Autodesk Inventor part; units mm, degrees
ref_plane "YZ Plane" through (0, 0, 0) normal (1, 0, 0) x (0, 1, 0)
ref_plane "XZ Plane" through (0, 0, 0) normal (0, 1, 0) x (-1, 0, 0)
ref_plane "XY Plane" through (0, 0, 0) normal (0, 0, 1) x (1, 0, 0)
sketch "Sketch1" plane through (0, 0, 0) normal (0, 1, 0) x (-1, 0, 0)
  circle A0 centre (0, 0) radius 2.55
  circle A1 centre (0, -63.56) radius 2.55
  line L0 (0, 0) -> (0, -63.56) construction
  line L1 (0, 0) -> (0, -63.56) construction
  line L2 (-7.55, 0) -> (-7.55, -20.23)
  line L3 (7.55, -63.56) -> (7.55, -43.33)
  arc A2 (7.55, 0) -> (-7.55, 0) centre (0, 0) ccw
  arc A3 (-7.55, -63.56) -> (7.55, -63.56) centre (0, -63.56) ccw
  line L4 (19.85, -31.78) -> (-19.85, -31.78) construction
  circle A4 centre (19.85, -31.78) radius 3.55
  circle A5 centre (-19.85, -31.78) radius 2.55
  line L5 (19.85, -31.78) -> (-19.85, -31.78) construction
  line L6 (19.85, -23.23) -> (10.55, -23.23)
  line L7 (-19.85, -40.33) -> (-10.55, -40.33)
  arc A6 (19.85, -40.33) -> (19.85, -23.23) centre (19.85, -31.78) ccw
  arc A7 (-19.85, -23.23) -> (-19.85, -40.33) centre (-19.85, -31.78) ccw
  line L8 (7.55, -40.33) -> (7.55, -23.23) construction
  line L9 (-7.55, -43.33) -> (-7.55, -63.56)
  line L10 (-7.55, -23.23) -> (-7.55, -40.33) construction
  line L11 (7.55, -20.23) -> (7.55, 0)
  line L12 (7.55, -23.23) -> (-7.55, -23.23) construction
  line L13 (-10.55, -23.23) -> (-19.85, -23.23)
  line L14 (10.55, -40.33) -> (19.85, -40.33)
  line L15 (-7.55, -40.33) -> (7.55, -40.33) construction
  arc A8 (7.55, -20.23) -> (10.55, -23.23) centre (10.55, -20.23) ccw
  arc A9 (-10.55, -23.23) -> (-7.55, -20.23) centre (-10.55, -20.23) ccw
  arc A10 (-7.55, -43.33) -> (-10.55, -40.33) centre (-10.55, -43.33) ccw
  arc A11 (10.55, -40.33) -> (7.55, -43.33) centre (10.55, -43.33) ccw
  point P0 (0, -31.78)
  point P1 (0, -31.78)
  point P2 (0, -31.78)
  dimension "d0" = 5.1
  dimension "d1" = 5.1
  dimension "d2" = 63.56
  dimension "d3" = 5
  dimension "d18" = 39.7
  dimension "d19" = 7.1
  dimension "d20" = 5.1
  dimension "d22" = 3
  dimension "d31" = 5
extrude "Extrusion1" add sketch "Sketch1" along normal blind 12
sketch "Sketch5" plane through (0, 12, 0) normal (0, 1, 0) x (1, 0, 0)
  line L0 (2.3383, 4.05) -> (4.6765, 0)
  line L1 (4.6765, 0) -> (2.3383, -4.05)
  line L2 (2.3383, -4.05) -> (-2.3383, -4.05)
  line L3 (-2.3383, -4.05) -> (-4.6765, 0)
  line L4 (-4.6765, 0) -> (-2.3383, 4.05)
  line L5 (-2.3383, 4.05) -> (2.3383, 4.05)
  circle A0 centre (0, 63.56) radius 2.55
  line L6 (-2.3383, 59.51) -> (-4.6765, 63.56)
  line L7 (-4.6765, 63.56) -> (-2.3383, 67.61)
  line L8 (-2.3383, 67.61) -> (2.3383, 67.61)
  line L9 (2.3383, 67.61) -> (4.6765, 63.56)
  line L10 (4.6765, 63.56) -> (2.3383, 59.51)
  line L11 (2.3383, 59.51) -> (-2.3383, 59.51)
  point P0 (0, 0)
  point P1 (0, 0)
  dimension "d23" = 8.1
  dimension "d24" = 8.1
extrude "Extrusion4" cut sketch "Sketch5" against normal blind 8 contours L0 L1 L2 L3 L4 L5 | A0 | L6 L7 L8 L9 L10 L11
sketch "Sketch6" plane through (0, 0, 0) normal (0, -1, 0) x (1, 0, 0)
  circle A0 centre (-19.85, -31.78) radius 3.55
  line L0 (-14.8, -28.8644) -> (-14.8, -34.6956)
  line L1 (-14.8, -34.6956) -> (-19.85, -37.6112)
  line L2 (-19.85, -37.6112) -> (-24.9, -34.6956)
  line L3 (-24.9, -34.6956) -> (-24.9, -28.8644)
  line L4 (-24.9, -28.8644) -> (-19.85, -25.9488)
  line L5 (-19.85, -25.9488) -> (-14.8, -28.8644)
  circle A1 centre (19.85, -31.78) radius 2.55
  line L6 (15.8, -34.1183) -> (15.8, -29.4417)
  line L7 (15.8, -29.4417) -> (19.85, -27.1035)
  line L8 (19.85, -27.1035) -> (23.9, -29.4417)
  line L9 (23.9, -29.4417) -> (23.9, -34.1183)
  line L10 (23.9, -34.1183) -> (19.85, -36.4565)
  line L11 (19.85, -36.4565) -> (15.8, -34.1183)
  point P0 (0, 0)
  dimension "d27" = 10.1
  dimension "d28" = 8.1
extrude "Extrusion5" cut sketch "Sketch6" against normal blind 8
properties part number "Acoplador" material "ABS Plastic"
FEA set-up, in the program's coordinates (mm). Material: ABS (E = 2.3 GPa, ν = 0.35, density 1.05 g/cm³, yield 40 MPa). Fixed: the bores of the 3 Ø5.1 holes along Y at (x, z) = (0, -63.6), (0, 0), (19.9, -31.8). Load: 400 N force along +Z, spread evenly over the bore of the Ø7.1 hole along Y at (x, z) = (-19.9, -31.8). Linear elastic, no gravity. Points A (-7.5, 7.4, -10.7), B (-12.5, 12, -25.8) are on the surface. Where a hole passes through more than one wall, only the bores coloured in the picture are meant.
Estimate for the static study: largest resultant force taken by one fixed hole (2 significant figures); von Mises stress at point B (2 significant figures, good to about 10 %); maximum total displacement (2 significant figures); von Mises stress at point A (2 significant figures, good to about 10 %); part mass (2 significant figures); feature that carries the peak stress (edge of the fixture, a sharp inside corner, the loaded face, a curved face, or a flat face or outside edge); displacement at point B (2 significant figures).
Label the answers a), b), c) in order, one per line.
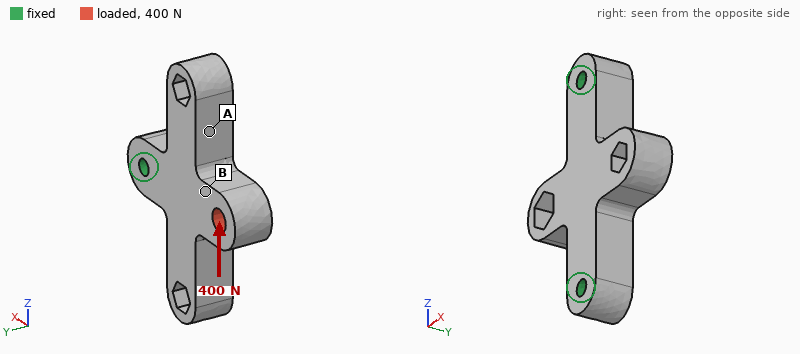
a) 270 N
b) 7.1 MPa
c) 0.27 mm
d) 3.2 MPa
e) 20 g
f) the loaded face
g) 0.092 mm
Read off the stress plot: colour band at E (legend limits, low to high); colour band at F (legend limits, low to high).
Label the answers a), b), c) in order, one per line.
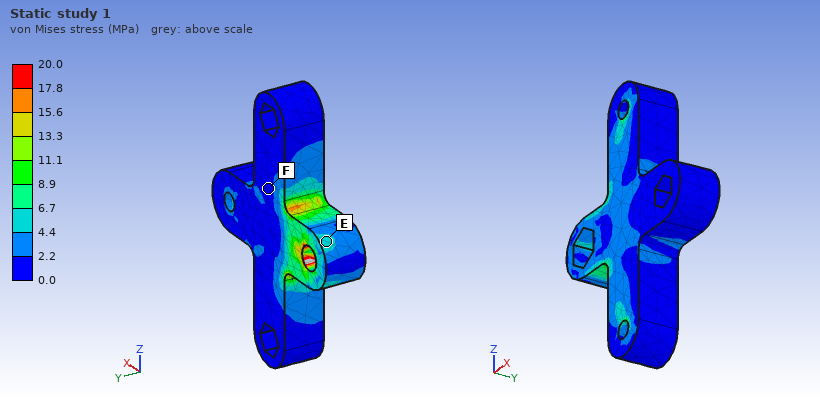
a) 4.4 to 6.7 MPa
b) 0.0 to 2.2 MPa
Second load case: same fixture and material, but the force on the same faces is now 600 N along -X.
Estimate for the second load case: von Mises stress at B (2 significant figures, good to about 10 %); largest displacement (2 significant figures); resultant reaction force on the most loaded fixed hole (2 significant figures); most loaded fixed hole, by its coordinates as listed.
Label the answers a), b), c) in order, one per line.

a) 9.9 MPa
b) 0.33 mm
c) 510 N
d) (19.9, -31.8)
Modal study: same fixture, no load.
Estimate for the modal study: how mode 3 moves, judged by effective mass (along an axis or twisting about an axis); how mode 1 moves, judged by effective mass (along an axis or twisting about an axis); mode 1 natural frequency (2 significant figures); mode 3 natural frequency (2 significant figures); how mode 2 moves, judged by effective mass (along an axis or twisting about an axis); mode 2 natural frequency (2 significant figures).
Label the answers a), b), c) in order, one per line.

a) along X
b) along Y
c) 1900 Hz
d) 5000 Hz
e) along Z
f) 4400 Hz
